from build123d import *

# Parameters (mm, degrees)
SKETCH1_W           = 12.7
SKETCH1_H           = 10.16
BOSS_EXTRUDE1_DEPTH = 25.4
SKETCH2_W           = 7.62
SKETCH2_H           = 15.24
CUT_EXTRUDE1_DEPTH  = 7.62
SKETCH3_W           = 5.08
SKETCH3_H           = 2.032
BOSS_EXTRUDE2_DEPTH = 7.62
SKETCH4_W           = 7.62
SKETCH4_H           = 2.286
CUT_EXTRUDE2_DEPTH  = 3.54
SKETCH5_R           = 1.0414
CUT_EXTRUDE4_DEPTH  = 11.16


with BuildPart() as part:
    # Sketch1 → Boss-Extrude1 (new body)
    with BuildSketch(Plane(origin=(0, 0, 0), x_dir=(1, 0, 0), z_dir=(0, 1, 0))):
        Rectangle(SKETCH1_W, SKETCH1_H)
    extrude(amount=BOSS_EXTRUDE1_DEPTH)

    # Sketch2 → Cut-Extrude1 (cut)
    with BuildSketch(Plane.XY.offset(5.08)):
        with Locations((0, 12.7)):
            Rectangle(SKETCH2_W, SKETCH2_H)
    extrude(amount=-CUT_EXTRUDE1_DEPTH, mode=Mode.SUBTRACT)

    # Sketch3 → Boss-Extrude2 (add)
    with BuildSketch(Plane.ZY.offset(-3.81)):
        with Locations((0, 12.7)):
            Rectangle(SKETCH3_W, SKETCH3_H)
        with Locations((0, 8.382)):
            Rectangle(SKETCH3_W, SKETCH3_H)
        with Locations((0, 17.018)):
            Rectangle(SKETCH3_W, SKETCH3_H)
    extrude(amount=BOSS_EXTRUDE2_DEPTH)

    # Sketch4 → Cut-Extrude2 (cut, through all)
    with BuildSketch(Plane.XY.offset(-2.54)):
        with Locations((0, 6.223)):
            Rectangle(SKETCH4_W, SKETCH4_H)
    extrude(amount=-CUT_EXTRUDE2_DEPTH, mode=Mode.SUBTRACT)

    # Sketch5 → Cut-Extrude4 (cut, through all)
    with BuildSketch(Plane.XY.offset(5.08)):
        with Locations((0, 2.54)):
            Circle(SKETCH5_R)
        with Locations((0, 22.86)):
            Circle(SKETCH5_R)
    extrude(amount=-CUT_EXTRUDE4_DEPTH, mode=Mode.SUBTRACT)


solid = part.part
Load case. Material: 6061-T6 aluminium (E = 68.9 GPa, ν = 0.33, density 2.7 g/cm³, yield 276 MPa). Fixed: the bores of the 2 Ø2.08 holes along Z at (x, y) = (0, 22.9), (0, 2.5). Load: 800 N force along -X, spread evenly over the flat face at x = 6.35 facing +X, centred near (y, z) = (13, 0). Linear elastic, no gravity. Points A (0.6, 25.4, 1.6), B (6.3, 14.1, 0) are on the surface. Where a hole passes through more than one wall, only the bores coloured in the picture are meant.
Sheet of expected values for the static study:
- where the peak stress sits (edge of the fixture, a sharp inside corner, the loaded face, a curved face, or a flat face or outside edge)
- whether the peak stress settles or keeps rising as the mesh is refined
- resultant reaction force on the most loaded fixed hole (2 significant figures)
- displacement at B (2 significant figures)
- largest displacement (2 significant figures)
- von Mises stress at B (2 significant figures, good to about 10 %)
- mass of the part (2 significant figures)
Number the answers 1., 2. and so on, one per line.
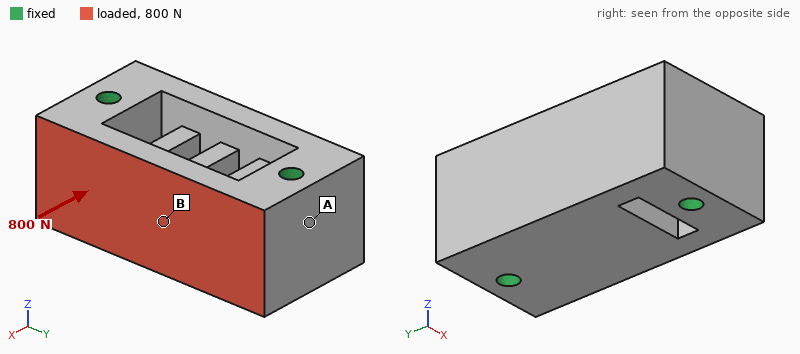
1. edge of the fixture
2. keeps rising
3. 410 N
4. 3.0 µm
5. 5.1 µm
6. 11 MPa
7. 6.8 g
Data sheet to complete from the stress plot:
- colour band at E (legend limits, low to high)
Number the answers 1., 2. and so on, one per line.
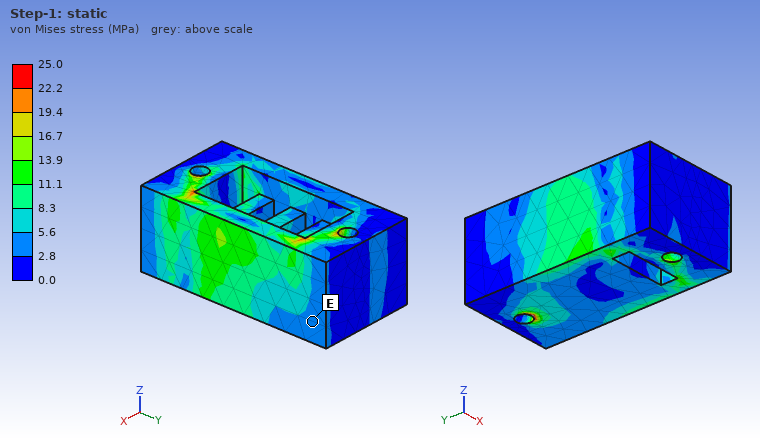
1. 2.8 to 5.6 MPa
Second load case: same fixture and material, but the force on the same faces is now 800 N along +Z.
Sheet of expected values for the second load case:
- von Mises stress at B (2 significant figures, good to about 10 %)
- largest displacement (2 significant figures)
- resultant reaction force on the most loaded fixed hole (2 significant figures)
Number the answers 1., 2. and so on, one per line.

1. 10.0 MPa
2. 7.3 µm
3. 410 N
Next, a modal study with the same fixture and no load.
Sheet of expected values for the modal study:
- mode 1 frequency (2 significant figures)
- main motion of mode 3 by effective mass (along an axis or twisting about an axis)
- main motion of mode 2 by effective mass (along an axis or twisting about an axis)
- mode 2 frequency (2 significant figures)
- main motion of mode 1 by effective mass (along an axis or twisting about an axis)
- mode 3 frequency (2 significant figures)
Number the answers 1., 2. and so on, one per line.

1. 38 kHz
2. twisting about Y
3. along Z
4. 42 kHz
5. along X
6. 49 kHz
